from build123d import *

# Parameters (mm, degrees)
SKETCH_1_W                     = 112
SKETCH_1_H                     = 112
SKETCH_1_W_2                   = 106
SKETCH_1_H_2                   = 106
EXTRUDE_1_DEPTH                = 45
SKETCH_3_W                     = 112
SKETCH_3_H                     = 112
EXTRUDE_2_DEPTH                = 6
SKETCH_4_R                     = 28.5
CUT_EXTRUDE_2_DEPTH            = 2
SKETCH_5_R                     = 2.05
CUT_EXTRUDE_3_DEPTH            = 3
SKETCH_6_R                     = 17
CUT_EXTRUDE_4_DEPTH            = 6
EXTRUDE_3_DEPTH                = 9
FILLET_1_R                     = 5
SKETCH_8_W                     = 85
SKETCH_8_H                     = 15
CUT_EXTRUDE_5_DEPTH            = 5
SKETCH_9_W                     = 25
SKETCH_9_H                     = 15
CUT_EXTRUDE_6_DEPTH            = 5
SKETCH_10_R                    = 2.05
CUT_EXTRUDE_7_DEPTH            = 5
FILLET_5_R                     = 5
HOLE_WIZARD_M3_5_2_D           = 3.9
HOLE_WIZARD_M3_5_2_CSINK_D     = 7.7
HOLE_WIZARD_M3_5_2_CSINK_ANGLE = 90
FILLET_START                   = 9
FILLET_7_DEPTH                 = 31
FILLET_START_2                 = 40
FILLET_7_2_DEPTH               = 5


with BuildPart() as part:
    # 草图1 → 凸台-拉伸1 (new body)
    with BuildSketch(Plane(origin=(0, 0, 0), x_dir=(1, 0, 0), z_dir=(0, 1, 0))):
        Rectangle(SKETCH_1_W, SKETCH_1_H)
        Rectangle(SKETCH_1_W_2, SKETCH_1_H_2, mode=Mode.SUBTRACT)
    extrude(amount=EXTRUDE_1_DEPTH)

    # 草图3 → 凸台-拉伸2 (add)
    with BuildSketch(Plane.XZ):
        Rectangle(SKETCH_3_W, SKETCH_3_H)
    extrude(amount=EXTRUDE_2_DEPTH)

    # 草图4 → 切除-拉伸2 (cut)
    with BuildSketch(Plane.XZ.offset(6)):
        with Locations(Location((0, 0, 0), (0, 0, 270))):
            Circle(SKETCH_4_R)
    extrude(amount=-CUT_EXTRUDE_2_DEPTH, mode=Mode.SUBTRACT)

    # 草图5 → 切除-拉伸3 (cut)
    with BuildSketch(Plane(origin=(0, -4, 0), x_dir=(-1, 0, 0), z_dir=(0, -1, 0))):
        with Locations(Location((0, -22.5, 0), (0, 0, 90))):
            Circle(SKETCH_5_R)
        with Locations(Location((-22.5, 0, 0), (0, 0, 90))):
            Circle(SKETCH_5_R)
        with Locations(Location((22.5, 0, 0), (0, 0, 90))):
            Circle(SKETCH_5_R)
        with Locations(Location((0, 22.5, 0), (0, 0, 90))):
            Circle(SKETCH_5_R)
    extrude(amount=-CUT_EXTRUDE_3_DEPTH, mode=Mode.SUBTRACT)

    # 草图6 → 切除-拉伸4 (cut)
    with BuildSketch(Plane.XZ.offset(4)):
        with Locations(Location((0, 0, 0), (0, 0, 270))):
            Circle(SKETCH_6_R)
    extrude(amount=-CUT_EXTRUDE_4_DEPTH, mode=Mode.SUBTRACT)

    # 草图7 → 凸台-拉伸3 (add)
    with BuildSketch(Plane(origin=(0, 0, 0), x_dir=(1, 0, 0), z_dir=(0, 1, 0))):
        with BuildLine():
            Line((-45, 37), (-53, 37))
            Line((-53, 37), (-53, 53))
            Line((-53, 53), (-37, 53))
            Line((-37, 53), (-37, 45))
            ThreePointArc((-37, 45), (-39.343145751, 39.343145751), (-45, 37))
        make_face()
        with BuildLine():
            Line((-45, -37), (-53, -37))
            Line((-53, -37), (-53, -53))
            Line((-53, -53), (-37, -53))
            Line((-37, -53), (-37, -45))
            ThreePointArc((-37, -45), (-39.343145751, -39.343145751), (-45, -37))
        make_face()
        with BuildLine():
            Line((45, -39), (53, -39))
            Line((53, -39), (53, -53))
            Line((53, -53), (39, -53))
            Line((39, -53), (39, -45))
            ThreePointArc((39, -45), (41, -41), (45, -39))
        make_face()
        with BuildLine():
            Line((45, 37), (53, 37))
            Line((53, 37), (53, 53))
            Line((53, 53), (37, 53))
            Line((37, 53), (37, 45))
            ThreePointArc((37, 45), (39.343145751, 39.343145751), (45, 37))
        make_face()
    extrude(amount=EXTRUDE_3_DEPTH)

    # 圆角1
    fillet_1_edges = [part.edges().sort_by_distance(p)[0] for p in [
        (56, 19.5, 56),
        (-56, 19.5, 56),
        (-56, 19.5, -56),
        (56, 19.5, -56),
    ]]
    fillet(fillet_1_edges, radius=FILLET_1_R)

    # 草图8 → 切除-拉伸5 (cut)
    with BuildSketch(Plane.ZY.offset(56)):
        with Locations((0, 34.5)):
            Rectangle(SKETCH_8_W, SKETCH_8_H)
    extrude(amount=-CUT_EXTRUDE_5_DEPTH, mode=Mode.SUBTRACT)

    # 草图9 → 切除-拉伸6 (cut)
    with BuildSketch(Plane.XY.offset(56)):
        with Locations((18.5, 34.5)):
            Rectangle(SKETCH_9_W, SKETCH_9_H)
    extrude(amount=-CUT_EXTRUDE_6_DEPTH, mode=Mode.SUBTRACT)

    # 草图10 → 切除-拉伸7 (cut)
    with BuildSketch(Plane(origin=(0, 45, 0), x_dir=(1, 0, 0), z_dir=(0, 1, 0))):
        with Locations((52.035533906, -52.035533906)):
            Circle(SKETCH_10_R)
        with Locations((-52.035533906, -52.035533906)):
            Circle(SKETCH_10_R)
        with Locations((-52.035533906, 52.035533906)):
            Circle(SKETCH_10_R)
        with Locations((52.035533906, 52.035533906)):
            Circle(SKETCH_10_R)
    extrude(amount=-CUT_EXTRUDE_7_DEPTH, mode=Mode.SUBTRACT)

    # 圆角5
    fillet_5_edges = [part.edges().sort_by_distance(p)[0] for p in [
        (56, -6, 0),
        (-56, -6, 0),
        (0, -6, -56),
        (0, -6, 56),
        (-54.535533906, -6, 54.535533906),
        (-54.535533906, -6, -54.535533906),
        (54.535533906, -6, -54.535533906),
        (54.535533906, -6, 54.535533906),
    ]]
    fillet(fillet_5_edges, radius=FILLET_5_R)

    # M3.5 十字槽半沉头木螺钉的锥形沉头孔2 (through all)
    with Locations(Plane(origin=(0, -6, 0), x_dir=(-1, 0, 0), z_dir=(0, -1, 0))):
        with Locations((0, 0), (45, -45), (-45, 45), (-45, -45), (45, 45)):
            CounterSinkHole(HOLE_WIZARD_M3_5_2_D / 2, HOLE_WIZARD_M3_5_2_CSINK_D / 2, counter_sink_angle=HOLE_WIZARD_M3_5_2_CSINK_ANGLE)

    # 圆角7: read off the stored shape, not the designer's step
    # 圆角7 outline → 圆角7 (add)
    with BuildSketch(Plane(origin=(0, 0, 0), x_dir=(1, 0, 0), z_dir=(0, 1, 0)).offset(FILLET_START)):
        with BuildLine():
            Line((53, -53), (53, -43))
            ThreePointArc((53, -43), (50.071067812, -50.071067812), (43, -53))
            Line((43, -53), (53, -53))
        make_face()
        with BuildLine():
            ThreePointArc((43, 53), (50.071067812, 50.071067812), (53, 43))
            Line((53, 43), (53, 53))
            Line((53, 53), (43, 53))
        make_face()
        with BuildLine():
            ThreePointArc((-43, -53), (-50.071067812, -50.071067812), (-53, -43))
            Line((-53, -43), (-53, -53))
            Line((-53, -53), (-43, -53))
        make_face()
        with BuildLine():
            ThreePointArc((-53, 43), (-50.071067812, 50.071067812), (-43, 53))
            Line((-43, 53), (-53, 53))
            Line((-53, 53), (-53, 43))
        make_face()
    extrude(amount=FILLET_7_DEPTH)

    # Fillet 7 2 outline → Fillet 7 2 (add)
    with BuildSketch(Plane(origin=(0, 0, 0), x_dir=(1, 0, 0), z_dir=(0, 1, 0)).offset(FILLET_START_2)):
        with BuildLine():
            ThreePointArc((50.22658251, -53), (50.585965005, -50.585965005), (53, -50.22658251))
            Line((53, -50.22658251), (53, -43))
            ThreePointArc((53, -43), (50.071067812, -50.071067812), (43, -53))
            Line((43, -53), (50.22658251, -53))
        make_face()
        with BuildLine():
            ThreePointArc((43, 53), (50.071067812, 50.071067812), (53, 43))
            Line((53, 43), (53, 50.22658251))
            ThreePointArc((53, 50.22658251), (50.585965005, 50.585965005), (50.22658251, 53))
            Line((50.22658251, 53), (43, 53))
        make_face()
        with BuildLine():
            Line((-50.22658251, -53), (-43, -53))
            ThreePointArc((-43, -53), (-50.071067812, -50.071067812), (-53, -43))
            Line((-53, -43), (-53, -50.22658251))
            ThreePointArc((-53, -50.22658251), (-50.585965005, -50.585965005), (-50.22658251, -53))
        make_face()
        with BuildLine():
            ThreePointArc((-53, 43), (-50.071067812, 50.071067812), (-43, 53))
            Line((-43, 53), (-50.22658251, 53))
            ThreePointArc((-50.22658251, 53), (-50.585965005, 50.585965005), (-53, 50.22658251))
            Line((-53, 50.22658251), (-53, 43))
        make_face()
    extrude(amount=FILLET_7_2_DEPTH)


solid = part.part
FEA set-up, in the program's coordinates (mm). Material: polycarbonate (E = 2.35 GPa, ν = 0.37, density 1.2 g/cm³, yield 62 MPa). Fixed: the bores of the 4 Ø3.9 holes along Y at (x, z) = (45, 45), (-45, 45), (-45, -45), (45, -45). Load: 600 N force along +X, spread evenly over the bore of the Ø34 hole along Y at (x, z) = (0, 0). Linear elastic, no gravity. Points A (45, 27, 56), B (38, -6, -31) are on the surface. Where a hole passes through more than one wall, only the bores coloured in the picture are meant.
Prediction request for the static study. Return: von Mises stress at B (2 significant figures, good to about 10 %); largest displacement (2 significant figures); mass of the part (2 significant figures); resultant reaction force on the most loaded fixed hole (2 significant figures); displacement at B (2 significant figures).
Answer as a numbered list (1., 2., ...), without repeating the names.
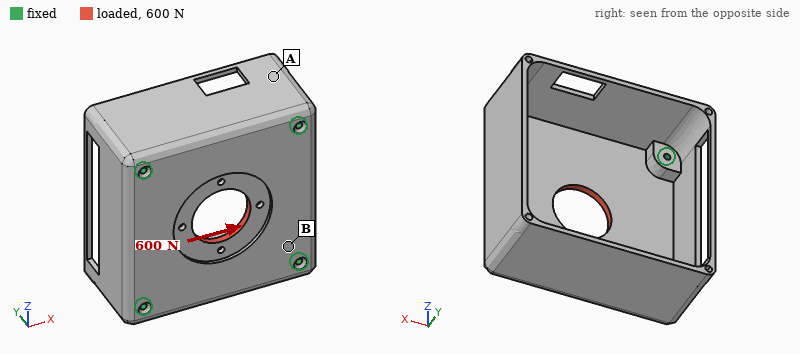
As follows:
1. 0.84 MPa
2. 40 µm
3. 150 g
4. 170 N
5. 13 µm
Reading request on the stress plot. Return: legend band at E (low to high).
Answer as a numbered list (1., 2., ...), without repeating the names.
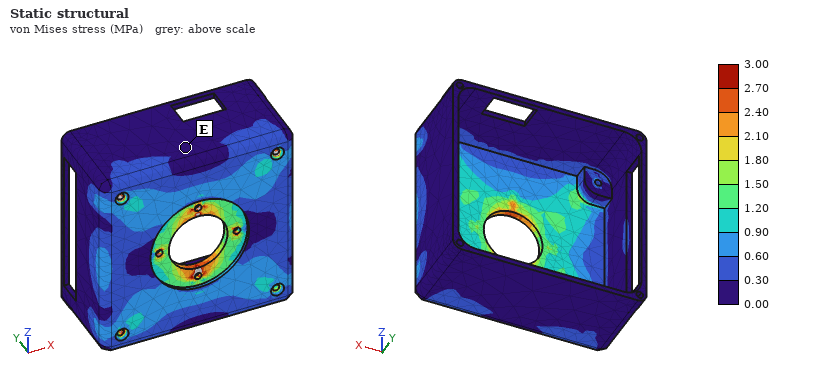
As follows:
1. 0.00 to 0.30 MPa
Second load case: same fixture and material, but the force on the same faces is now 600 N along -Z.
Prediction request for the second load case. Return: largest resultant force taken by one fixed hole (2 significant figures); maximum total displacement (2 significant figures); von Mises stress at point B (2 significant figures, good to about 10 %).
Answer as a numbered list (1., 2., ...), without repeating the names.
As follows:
1. 170 N
2. 40 µm
3. 0.90 MPa
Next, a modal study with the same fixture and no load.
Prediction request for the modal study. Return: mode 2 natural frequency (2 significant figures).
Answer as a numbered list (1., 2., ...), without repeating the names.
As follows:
1. 560 Hz
